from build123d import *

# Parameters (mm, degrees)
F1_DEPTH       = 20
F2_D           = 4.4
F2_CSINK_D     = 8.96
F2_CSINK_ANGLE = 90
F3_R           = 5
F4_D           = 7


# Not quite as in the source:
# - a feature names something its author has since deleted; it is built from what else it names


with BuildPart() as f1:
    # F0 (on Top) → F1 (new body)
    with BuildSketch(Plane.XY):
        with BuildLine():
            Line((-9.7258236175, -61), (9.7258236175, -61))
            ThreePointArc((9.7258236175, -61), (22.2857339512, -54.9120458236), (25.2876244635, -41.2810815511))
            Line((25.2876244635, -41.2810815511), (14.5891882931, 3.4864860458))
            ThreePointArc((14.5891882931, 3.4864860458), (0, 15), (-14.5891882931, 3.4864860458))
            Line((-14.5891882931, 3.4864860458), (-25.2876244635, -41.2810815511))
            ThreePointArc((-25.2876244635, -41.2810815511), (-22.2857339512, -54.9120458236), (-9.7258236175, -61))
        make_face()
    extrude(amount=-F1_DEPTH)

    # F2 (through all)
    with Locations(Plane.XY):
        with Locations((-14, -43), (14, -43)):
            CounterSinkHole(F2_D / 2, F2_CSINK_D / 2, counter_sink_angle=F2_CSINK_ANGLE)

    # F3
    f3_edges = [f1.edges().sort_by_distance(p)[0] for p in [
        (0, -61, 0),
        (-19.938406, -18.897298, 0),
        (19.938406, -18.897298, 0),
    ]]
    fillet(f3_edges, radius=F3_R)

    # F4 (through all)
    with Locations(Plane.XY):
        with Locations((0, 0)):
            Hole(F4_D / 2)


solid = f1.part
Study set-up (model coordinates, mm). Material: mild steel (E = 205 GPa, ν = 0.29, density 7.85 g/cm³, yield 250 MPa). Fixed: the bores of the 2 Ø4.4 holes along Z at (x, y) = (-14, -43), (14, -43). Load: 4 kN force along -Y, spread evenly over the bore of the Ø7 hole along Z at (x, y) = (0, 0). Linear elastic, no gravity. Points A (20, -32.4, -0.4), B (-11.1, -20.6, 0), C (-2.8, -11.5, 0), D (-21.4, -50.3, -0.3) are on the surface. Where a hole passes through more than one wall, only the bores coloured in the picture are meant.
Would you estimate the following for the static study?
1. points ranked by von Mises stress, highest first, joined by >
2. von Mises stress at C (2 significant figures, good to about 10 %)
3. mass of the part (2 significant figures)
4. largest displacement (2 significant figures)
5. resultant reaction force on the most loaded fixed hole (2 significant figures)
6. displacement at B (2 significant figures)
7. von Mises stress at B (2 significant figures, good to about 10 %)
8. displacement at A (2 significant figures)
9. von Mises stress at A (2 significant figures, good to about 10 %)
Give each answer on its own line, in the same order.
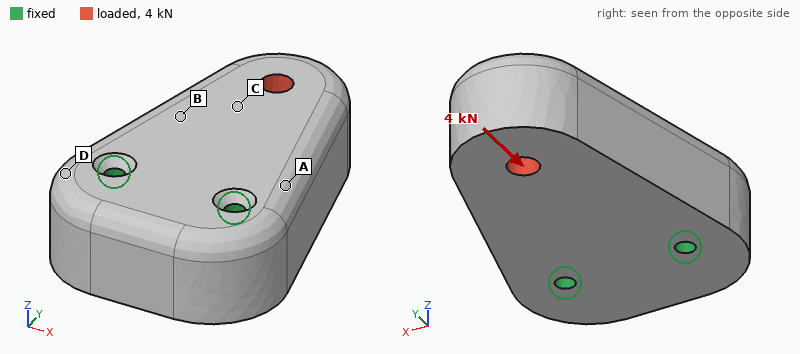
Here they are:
C > B > A > D
7.6 MPa
440 g
1.8 µm
2.0 kN
0.71 µm
5.4 MPa
0.39 µm
3.7 MPa
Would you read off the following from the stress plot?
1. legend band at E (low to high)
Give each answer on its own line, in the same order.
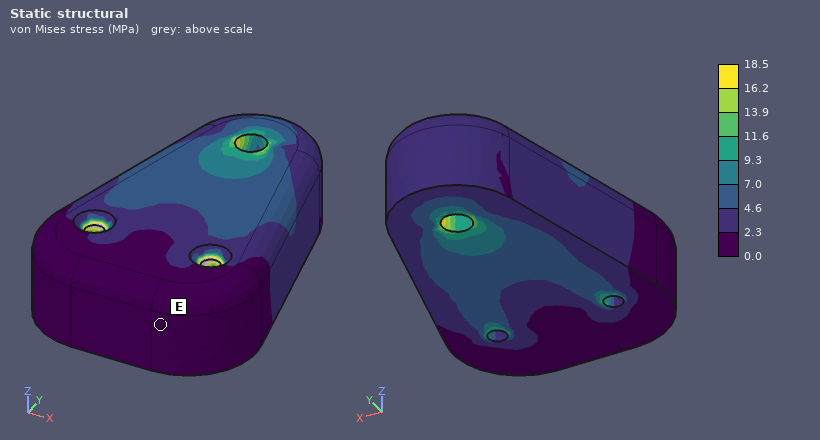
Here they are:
0.0 to 2.3 MPa
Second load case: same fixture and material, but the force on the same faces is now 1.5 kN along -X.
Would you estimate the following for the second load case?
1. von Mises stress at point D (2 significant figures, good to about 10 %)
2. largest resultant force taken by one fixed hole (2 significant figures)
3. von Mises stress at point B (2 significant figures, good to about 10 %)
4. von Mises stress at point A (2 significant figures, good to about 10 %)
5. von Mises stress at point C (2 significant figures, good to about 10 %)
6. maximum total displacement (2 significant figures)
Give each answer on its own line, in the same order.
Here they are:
2.3 MPa
2.3 kN
4.2 MPa
5.0 MPa
4.8 MPa
3.7 µm
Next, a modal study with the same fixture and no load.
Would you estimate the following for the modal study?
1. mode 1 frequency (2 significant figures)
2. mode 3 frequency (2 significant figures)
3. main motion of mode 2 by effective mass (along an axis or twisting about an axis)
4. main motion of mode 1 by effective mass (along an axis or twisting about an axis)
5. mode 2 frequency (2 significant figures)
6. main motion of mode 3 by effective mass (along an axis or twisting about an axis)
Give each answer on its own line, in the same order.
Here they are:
5200 Hz
15 kHz
along X
along Z
9800 Hz
twisting about Y
